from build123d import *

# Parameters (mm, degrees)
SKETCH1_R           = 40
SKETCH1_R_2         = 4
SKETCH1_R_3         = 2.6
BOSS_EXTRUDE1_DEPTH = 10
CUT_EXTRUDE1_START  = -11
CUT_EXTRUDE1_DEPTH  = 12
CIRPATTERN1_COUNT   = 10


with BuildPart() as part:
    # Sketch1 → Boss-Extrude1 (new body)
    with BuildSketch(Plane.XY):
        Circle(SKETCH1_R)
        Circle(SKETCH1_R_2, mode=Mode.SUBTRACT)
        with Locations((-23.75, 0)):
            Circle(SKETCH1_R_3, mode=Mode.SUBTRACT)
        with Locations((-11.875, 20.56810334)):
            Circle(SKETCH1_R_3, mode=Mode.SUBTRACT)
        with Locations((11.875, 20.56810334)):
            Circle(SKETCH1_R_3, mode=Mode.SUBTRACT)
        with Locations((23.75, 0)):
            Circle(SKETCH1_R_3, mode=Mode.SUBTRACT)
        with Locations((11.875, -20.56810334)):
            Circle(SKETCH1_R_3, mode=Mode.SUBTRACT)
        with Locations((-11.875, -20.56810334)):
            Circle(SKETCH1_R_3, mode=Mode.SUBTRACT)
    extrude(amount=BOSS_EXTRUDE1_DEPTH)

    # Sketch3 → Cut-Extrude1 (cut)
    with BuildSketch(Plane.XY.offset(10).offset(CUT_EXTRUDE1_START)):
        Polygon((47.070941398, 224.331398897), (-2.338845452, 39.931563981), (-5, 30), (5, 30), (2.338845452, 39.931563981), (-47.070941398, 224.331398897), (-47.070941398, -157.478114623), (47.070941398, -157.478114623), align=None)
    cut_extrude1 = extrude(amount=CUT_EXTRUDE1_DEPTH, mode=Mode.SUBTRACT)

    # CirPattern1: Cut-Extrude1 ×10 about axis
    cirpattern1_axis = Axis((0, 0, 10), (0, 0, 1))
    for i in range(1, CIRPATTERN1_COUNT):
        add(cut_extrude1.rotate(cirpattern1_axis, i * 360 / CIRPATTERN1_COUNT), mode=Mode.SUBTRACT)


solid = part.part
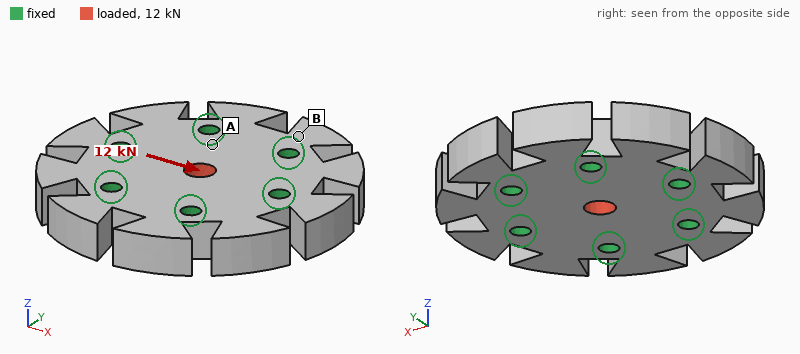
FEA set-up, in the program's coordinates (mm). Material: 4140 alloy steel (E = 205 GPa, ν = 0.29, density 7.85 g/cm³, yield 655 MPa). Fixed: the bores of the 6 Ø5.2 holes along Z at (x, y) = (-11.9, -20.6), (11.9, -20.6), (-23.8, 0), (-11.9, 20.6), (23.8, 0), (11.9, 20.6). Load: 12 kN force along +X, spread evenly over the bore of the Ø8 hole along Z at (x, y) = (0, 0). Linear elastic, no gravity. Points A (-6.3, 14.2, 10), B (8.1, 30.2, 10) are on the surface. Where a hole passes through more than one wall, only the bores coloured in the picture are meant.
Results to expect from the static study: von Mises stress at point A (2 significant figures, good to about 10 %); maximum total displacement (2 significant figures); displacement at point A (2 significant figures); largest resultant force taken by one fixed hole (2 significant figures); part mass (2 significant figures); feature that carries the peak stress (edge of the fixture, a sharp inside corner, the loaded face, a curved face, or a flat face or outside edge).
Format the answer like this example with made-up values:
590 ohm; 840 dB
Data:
14 MPa; 2.9 µm; 0.53 µm; 3.2 kN; 320 g; the loaded face
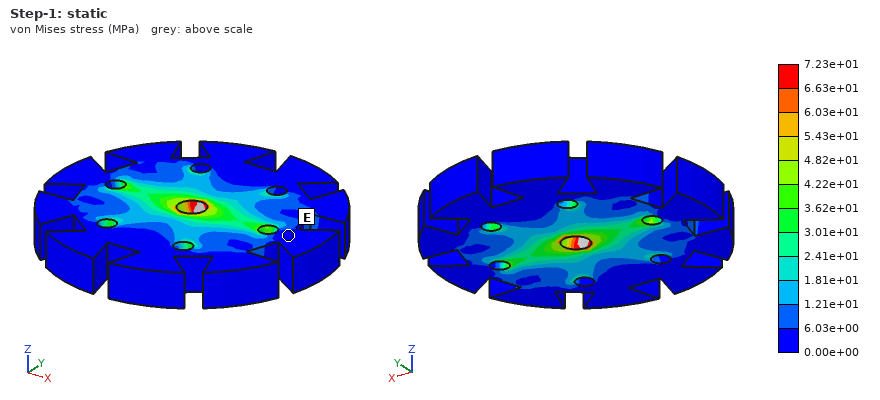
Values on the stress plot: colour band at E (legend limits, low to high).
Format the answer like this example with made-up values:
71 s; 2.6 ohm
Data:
0.00e+00 to 6.03e+00 MPa
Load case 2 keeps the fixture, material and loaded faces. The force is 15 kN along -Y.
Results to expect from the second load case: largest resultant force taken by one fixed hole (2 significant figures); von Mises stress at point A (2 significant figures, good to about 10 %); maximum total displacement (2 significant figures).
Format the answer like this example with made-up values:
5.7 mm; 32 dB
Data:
3.5 kN; 31 MPa; 3.7 µm
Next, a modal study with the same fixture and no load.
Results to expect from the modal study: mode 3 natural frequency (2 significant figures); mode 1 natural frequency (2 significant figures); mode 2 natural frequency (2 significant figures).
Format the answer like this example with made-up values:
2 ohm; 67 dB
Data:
18 kHz; 18 kHz; 18 kHz
